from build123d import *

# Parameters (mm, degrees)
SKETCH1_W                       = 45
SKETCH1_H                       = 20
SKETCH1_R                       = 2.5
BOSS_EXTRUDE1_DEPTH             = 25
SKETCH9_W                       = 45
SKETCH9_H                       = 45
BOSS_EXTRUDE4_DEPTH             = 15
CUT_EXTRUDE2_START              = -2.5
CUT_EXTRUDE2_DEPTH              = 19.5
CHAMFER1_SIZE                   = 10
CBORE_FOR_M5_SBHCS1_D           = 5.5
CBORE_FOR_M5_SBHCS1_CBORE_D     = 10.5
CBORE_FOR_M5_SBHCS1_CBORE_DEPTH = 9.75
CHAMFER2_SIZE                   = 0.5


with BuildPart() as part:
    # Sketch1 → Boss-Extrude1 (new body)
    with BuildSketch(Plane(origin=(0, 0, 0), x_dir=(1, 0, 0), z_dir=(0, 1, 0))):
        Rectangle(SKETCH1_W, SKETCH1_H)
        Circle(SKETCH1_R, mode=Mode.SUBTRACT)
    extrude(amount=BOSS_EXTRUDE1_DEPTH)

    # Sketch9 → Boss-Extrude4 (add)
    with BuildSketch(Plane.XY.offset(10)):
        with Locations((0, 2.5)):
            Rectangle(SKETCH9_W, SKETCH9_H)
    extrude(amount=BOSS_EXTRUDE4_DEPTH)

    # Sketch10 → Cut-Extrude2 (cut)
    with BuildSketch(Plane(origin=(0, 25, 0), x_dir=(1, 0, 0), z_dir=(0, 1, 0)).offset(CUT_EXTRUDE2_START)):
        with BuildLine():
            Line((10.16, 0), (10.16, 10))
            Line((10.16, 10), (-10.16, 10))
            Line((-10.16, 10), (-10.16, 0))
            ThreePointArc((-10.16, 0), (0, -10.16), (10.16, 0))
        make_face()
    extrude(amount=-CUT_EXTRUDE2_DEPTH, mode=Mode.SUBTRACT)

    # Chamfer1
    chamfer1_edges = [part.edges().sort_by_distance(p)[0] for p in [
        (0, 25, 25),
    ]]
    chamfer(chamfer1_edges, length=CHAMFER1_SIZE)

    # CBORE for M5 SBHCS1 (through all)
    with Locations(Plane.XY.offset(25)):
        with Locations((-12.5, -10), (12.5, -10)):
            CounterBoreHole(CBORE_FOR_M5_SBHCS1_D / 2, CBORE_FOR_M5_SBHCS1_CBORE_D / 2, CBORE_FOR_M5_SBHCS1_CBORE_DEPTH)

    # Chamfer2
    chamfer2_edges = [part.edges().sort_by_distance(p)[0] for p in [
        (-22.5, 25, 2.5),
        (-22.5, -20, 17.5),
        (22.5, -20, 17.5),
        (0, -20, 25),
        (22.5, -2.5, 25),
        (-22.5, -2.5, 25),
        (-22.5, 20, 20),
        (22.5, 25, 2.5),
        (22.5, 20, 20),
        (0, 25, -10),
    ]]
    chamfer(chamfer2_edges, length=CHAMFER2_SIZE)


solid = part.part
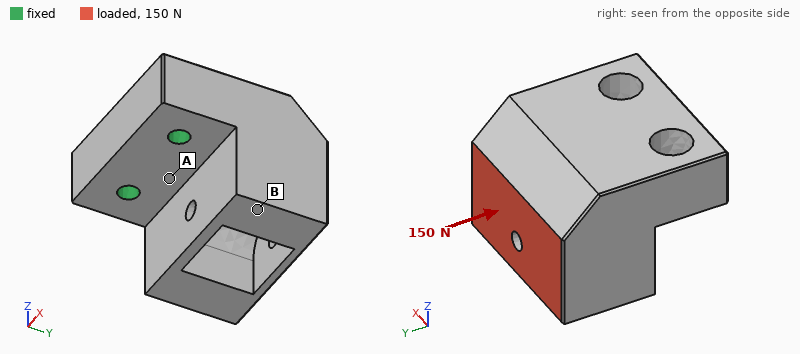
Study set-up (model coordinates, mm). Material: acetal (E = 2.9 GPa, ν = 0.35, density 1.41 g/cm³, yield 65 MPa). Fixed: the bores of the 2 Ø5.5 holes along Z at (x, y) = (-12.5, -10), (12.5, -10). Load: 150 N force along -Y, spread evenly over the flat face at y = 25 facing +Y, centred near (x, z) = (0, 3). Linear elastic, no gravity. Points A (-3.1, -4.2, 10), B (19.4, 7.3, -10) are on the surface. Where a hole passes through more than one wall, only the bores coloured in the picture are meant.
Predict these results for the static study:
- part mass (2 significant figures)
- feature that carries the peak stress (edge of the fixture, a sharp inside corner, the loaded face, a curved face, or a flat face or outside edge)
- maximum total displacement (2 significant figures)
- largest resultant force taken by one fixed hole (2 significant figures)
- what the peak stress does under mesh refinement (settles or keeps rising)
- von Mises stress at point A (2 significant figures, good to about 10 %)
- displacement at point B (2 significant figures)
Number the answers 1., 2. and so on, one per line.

1. 58 g
2. edge of the fixture
3. 0.14 mm
4. 76 N
5. keeps rising
6. 1.2 MPa
7. 0.081 mm
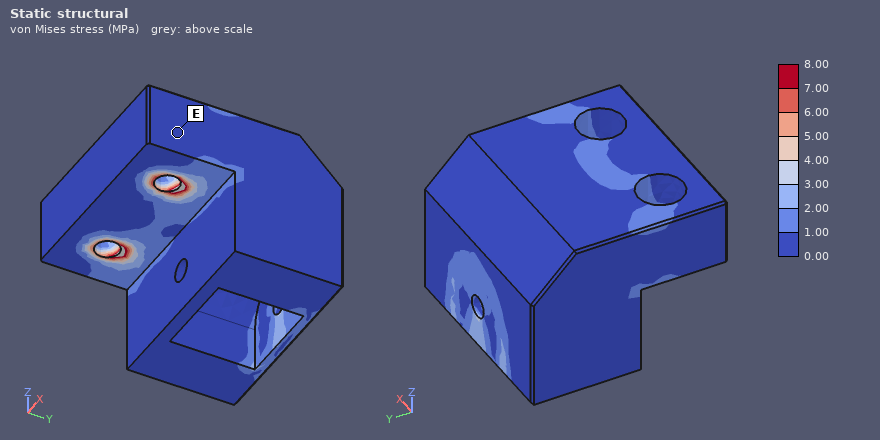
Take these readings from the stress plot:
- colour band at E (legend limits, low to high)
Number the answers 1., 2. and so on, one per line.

1. 0.00 to 1.00 MPa
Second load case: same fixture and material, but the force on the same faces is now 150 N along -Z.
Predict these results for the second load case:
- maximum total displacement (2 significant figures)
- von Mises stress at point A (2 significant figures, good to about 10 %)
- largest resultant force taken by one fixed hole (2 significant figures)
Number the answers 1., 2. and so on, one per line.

1. 0.35 mm
2. 2.8 MPa
3. 78 N
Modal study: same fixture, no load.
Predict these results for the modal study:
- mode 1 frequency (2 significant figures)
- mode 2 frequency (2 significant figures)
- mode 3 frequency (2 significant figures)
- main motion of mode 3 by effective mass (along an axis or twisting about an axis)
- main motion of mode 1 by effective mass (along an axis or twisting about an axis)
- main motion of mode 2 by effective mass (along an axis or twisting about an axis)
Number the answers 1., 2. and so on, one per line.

1. 780 Hz
2. 1800 Hz
3. 2700 Hz
4. along X
5. along Z
6. along X
